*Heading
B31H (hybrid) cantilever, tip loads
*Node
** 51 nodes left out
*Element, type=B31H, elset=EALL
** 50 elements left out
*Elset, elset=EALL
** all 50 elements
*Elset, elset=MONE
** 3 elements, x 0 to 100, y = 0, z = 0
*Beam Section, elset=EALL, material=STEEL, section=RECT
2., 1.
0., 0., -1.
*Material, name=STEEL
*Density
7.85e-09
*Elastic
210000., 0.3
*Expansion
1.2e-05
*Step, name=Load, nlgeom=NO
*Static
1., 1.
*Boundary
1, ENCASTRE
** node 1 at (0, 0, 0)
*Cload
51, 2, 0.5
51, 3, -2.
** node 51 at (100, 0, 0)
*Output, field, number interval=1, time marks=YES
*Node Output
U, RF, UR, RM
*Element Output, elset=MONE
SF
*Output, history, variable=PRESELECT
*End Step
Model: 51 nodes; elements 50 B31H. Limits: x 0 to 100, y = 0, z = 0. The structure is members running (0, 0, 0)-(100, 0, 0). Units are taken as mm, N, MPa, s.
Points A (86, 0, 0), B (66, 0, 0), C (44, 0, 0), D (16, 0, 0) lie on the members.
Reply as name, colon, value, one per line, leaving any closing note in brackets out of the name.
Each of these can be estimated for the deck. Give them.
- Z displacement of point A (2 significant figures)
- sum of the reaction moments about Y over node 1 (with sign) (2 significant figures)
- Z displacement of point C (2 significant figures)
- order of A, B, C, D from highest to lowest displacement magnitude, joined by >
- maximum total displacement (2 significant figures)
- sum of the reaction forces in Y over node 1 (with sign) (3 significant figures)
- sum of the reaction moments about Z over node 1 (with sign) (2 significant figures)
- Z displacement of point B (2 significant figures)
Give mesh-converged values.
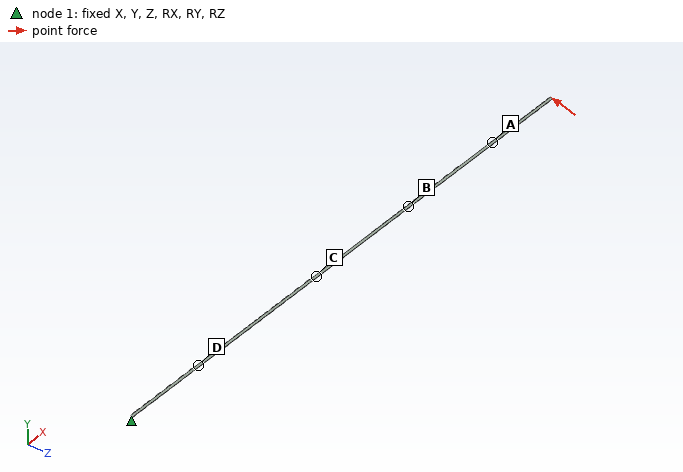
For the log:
Z displacement of point A: -3.8 mm
sum of the reaction moments about Y over node 1 (with sign): -200 N·mm
Z displacement of point C: -1.2 mm
order of A, B, C, D from highest to lowest displacement magnitude, joined by >: A > B > C > D
maximum total displacement: 6.7 mm
sum of the reaction forces in Y over node 1 (with sign): -0.500 N
sum of the reaction moments about Z over node 1 (with sign): -50 N·mm
Z displacement of point B: -2.4 mm
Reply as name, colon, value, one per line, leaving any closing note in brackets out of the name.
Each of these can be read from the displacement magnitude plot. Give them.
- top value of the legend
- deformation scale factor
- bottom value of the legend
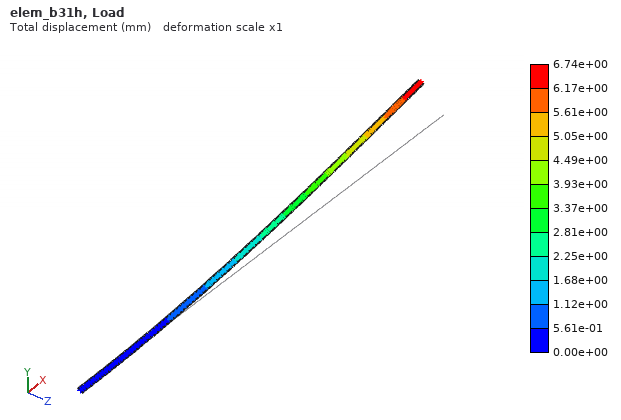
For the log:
top value of the legend: 6.74e+00 mm
deformation scale factor: 1
bottom value of the legend: 0.00e+00 mm
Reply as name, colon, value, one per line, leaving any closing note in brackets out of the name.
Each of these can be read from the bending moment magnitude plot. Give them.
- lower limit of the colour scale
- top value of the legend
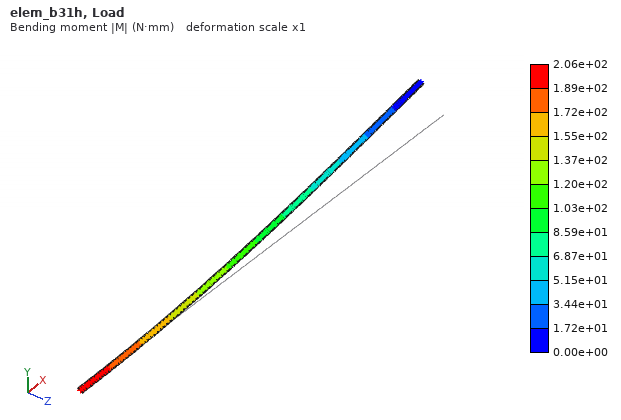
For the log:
lower limit of the colour scale: 0.00e+00 N·mm
top value of the legend: 2.06e+02 N·mm
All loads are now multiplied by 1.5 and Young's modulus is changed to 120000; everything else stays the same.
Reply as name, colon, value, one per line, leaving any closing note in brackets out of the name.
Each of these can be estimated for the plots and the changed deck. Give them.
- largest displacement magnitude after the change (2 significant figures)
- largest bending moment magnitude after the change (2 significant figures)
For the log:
largest displacement magnitude after the change: 18 mm
largest bending moment magnitude after the change: 310 N·mm
